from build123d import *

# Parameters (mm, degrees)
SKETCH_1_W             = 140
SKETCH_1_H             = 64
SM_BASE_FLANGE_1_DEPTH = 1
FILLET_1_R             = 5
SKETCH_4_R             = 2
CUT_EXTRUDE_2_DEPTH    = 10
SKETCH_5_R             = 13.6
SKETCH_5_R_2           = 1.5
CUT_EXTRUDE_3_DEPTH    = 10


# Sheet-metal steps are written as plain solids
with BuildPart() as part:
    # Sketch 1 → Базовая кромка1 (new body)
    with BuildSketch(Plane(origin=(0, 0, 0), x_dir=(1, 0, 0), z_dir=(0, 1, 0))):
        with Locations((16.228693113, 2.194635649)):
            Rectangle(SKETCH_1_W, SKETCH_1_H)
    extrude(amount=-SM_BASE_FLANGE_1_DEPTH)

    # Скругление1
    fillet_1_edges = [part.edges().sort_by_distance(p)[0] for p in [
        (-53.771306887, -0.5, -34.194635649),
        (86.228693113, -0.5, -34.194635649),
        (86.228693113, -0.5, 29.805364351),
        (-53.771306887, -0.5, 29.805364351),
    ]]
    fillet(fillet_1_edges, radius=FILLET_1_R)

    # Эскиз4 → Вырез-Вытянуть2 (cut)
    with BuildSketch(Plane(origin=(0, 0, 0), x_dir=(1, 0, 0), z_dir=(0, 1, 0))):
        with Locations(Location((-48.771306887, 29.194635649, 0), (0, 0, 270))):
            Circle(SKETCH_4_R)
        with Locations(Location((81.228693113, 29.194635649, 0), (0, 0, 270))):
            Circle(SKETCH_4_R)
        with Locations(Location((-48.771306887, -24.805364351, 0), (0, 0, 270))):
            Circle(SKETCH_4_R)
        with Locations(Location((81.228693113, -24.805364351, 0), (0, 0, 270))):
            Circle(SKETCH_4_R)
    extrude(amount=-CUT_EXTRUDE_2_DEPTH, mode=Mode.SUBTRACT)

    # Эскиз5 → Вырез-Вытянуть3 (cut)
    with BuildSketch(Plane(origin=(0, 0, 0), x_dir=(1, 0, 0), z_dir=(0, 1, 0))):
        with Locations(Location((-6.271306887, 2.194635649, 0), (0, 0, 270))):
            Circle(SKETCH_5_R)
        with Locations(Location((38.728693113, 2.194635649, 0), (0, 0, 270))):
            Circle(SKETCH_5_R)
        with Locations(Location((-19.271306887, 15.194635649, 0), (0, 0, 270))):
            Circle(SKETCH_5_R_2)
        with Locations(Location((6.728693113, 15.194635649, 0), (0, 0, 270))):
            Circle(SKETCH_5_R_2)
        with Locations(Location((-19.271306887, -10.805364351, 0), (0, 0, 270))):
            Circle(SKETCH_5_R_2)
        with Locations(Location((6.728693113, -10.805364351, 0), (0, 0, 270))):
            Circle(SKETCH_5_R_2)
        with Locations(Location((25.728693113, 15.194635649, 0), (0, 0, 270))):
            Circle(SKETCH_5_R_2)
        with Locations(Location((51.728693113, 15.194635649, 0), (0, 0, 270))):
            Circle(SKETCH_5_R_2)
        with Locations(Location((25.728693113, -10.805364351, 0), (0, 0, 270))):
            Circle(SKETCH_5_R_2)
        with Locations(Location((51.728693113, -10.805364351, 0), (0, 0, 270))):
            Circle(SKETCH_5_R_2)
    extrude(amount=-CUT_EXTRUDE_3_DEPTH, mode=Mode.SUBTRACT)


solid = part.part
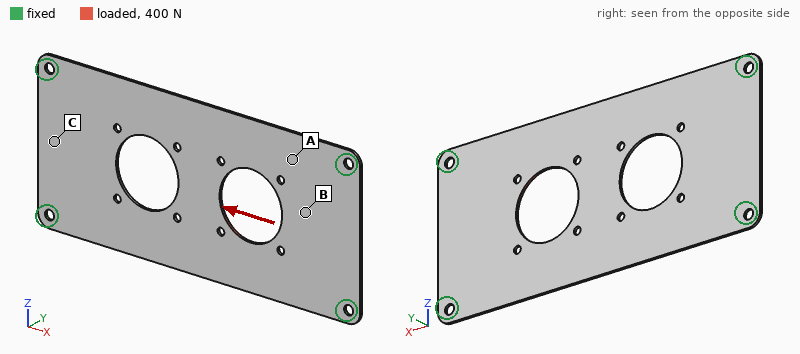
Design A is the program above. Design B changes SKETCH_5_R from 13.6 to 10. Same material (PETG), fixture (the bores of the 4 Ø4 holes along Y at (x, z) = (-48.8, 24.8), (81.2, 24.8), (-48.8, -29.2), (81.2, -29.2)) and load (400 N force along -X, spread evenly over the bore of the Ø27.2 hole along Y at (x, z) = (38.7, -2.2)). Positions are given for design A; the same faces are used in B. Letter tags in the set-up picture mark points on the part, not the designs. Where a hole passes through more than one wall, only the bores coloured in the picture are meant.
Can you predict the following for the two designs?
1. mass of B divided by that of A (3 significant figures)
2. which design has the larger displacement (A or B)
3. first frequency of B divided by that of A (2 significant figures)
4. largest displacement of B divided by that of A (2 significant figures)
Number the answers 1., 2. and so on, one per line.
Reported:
1. 1.07
2. A
3. 0.98
4. 0.92
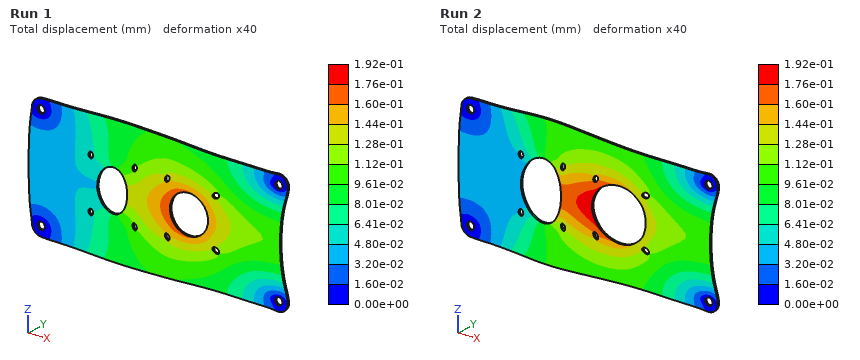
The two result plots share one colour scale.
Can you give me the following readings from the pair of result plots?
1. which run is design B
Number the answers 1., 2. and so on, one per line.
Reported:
1. Run 1
